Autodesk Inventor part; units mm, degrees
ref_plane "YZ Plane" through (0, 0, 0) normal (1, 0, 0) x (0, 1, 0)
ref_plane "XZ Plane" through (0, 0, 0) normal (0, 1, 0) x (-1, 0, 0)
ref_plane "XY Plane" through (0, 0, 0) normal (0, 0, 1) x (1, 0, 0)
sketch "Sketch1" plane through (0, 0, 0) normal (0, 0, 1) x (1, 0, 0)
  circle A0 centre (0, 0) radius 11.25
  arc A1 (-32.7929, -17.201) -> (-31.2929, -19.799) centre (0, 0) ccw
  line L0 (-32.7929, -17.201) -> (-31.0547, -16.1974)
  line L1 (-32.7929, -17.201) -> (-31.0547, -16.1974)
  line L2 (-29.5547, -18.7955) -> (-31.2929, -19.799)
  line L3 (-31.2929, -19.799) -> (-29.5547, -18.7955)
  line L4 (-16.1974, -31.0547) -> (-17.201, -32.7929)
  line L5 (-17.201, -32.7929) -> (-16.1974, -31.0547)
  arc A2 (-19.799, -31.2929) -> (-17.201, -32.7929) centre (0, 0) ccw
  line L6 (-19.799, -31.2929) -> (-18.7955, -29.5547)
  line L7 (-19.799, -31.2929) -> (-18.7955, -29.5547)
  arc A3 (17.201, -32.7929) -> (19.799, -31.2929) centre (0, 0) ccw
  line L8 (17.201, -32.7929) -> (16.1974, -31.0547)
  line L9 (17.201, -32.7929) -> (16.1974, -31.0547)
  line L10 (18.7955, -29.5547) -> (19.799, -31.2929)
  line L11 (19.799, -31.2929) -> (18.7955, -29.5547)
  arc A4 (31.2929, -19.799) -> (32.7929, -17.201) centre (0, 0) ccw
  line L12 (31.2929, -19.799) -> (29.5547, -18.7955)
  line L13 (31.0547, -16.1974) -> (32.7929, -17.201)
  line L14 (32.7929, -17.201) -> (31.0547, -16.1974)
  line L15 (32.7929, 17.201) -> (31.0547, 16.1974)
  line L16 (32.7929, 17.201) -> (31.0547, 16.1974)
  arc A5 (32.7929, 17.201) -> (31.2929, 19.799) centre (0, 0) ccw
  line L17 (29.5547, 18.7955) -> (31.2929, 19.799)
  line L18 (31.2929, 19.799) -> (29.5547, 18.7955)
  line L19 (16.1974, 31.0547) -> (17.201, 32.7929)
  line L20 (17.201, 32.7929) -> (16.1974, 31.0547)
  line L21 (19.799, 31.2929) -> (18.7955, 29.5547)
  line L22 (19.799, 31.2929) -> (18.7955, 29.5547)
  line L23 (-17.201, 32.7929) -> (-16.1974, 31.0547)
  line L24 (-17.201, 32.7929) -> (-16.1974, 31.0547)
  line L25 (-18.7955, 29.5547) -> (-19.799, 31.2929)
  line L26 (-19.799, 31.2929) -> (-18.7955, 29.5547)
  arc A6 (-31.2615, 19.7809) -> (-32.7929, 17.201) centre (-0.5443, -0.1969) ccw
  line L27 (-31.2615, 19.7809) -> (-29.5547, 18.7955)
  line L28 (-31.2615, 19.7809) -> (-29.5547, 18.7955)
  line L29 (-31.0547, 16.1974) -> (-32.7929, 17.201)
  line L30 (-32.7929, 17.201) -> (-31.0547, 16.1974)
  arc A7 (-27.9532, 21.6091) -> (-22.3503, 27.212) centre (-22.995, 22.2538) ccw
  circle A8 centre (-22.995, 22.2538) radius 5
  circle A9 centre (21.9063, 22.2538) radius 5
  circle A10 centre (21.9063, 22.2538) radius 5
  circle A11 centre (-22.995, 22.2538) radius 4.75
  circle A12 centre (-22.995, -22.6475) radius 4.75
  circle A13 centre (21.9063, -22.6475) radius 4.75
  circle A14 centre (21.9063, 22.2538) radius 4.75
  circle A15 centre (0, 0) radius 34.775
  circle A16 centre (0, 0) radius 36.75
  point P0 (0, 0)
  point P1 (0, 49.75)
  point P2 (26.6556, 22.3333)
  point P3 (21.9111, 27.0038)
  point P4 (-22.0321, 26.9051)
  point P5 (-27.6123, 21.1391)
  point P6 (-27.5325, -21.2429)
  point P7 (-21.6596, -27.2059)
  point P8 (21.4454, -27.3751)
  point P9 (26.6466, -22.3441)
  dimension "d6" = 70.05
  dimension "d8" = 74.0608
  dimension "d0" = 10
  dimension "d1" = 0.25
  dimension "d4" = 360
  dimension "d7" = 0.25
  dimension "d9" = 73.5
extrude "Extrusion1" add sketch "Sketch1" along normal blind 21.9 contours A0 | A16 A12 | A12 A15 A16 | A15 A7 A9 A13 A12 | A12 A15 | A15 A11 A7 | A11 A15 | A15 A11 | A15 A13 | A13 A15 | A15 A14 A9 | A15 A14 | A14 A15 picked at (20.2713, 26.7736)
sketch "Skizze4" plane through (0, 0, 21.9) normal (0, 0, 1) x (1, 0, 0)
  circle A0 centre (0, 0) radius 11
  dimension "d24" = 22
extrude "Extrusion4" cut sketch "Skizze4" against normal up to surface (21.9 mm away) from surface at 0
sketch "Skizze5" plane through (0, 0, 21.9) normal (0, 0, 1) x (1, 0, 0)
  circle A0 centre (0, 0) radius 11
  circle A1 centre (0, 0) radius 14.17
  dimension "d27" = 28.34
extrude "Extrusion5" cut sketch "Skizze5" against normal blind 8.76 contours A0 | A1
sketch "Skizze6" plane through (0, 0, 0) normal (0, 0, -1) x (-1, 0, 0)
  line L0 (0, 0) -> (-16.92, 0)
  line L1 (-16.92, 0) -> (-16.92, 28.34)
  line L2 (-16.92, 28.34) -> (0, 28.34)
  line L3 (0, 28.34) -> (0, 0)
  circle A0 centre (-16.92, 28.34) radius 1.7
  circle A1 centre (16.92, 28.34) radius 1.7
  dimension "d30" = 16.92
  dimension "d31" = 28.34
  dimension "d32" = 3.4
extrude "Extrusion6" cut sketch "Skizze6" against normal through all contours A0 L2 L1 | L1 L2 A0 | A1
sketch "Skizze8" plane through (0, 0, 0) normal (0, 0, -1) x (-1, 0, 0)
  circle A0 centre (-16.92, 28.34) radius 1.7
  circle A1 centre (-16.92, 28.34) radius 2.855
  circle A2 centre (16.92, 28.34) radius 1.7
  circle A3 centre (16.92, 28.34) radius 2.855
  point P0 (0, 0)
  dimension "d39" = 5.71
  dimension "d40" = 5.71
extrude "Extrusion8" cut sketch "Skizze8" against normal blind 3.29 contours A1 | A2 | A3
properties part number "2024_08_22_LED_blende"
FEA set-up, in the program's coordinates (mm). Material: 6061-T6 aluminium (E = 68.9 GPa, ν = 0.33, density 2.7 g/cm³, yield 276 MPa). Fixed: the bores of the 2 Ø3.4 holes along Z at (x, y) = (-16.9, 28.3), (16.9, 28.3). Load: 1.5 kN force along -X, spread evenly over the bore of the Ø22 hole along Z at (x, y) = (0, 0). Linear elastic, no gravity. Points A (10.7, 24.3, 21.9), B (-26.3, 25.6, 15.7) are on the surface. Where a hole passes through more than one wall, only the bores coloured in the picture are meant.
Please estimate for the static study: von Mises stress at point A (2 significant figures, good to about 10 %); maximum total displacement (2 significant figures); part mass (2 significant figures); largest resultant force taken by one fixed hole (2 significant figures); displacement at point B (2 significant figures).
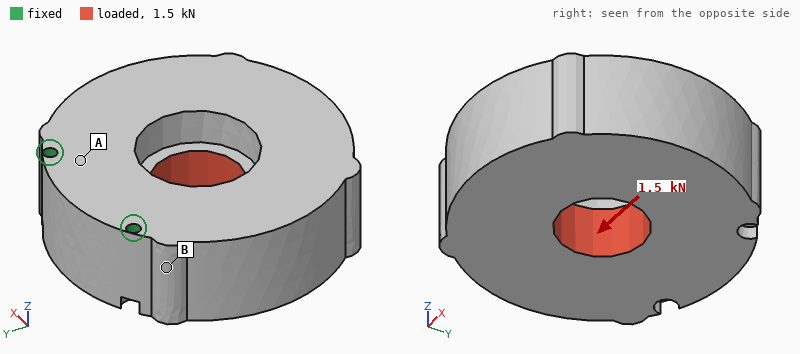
4.1 MPa
8.9 µm
200 g
1.4 kN
2.2 µm
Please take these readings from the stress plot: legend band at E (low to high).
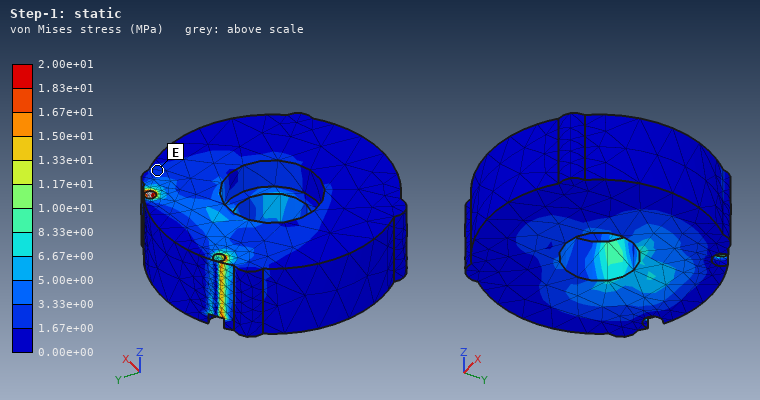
1.67e+00 to 3.33e+00 MPa
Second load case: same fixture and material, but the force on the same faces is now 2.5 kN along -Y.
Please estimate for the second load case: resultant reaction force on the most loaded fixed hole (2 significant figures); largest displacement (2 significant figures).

1.3 kN
12 µm
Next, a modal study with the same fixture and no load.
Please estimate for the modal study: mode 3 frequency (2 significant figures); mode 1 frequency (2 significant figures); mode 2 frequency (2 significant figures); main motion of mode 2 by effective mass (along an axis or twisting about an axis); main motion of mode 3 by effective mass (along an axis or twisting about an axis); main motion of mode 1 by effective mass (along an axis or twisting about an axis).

7300 Hz
3000 Hz
5100 Hz
along X
twisting about Y
along Z
